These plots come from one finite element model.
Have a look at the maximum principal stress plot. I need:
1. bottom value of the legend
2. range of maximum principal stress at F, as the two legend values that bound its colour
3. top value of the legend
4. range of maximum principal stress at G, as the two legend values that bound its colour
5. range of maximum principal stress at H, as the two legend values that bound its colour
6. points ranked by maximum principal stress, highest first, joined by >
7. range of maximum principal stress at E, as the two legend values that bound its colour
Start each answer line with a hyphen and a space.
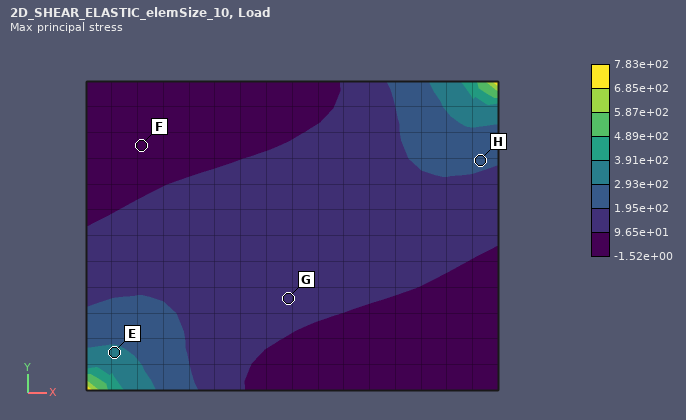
- -1.52e+00
- -1.52e+00 to 9.65e+01
- 7.83e+02
- 9.65e+01 to 1.95e+02
- 1.95e+02 to 2.93e+02
- E > H > G > F
- 2.93e+02 to 3.91e+02
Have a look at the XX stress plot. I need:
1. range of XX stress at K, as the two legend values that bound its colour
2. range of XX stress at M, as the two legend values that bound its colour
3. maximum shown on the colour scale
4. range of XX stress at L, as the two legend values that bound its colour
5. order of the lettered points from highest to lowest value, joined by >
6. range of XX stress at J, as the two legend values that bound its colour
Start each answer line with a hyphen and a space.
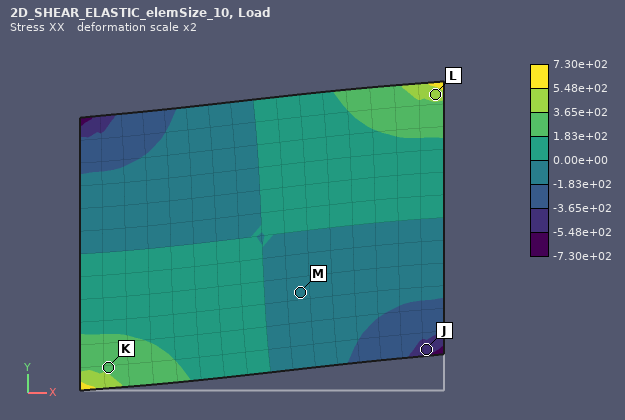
- 1.83e+02 to 3.65e+02
- -1.83e+02 to 0.00e+00
- 7.30e+02
- 3.65e+02 to 5.48e+02
- L > K > M > J
- -5.48e+02 to -3.65e+02
